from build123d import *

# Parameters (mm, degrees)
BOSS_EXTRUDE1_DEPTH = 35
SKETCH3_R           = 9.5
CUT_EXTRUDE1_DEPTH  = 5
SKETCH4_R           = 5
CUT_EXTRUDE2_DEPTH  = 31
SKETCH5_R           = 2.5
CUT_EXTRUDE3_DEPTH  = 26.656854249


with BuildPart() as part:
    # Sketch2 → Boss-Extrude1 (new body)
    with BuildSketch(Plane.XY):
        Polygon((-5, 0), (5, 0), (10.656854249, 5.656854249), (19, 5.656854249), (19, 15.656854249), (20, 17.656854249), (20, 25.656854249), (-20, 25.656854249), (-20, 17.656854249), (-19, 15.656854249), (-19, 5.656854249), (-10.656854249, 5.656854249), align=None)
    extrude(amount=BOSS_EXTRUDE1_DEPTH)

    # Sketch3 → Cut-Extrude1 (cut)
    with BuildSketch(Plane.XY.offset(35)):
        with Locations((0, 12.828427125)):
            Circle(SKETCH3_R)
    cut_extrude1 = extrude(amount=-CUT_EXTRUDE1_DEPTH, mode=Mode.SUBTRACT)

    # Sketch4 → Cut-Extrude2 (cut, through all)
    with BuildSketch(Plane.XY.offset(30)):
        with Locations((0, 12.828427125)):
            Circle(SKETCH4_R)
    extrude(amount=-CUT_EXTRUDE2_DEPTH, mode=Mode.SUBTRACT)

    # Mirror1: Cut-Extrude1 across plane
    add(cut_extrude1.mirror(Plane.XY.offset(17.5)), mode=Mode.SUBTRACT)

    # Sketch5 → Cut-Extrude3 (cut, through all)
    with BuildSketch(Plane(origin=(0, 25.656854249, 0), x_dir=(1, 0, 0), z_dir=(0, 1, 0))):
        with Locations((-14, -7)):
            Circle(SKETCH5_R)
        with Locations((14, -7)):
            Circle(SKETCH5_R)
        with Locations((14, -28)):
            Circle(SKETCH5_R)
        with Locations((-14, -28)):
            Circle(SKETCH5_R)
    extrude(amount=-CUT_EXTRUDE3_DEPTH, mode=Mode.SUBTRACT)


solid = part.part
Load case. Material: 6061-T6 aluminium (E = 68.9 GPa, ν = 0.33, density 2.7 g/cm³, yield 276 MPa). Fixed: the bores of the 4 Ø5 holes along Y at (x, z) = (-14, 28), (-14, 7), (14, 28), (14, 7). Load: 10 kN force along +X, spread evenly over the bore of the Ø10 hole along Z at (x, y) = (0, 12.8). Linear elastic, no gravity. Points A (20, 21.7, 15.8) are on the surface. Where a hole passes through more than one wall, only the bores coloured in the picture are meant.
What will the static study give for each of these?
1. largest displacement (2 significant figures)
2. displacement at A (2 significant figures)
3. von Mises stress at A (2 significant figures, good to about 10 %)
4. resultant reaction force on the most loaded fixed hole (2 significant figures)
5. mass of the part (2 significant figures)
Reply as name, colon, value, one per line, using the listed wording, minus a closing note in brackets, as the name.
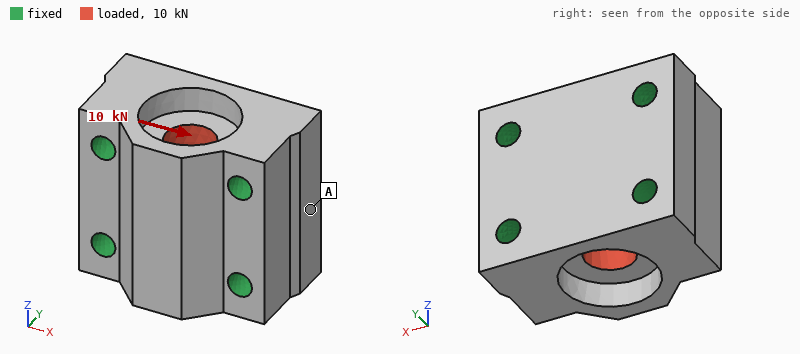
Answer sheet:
largest displacement: 3.1 µm
displacement at A: 0.83 µm
von Mises stress at A: 4.8 MPa
resultant reaction force on the most loaded fixed hole: 2.6 kN
mass of the part: 65 g
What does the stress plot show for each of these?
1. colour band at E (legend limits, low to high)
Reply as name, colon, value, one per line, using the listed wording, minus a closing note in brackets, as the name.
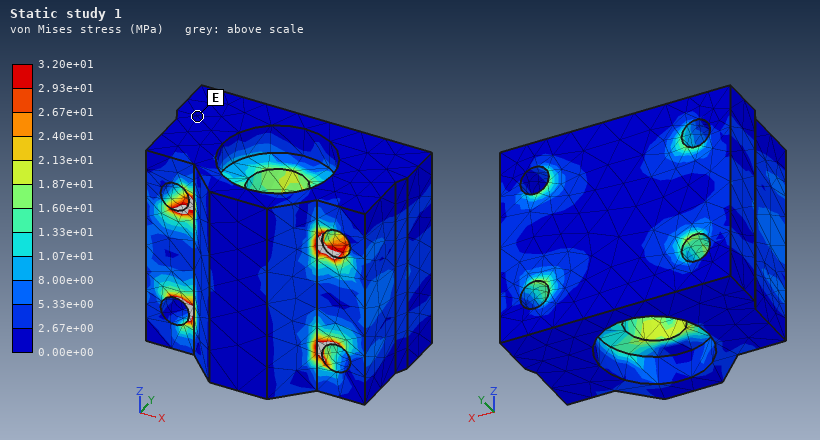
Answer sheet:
colour band at E: 0.00e+00 to 2.67e+00 MPa
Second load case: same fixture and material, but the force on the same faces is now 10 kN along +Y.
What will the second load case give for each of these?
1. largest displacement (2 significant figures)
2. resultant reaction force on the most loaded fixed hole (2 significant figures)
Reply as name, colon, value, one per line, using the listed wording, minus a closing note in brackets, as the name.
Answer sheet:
largest displacement: 5.5 µm
resultant reaction force on the most loaded fixed hole: 2.5 kN
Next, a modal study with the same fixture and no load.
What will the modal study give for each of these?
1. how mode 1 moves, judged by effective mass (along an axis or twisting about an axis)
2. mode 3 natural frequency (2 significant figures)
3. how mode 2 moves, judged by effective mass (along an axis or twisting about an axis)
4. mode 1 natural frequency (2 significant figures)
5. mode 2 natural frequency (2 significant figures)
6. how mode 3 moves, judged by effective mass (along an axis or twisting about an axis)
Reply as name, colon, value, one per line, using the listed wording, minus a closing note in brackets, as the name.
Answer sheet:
how mode 1 moves, judged by effective mass: along Z
mode 3 natural frequency: 57 kHz
how mode 2 moves, judged by effective mass: along Y
mode 1 natural frequency: 44 kHz
mode 2 natural frequency: 49 kHz
how mode 3 moves, judged by effective mass: along Z
